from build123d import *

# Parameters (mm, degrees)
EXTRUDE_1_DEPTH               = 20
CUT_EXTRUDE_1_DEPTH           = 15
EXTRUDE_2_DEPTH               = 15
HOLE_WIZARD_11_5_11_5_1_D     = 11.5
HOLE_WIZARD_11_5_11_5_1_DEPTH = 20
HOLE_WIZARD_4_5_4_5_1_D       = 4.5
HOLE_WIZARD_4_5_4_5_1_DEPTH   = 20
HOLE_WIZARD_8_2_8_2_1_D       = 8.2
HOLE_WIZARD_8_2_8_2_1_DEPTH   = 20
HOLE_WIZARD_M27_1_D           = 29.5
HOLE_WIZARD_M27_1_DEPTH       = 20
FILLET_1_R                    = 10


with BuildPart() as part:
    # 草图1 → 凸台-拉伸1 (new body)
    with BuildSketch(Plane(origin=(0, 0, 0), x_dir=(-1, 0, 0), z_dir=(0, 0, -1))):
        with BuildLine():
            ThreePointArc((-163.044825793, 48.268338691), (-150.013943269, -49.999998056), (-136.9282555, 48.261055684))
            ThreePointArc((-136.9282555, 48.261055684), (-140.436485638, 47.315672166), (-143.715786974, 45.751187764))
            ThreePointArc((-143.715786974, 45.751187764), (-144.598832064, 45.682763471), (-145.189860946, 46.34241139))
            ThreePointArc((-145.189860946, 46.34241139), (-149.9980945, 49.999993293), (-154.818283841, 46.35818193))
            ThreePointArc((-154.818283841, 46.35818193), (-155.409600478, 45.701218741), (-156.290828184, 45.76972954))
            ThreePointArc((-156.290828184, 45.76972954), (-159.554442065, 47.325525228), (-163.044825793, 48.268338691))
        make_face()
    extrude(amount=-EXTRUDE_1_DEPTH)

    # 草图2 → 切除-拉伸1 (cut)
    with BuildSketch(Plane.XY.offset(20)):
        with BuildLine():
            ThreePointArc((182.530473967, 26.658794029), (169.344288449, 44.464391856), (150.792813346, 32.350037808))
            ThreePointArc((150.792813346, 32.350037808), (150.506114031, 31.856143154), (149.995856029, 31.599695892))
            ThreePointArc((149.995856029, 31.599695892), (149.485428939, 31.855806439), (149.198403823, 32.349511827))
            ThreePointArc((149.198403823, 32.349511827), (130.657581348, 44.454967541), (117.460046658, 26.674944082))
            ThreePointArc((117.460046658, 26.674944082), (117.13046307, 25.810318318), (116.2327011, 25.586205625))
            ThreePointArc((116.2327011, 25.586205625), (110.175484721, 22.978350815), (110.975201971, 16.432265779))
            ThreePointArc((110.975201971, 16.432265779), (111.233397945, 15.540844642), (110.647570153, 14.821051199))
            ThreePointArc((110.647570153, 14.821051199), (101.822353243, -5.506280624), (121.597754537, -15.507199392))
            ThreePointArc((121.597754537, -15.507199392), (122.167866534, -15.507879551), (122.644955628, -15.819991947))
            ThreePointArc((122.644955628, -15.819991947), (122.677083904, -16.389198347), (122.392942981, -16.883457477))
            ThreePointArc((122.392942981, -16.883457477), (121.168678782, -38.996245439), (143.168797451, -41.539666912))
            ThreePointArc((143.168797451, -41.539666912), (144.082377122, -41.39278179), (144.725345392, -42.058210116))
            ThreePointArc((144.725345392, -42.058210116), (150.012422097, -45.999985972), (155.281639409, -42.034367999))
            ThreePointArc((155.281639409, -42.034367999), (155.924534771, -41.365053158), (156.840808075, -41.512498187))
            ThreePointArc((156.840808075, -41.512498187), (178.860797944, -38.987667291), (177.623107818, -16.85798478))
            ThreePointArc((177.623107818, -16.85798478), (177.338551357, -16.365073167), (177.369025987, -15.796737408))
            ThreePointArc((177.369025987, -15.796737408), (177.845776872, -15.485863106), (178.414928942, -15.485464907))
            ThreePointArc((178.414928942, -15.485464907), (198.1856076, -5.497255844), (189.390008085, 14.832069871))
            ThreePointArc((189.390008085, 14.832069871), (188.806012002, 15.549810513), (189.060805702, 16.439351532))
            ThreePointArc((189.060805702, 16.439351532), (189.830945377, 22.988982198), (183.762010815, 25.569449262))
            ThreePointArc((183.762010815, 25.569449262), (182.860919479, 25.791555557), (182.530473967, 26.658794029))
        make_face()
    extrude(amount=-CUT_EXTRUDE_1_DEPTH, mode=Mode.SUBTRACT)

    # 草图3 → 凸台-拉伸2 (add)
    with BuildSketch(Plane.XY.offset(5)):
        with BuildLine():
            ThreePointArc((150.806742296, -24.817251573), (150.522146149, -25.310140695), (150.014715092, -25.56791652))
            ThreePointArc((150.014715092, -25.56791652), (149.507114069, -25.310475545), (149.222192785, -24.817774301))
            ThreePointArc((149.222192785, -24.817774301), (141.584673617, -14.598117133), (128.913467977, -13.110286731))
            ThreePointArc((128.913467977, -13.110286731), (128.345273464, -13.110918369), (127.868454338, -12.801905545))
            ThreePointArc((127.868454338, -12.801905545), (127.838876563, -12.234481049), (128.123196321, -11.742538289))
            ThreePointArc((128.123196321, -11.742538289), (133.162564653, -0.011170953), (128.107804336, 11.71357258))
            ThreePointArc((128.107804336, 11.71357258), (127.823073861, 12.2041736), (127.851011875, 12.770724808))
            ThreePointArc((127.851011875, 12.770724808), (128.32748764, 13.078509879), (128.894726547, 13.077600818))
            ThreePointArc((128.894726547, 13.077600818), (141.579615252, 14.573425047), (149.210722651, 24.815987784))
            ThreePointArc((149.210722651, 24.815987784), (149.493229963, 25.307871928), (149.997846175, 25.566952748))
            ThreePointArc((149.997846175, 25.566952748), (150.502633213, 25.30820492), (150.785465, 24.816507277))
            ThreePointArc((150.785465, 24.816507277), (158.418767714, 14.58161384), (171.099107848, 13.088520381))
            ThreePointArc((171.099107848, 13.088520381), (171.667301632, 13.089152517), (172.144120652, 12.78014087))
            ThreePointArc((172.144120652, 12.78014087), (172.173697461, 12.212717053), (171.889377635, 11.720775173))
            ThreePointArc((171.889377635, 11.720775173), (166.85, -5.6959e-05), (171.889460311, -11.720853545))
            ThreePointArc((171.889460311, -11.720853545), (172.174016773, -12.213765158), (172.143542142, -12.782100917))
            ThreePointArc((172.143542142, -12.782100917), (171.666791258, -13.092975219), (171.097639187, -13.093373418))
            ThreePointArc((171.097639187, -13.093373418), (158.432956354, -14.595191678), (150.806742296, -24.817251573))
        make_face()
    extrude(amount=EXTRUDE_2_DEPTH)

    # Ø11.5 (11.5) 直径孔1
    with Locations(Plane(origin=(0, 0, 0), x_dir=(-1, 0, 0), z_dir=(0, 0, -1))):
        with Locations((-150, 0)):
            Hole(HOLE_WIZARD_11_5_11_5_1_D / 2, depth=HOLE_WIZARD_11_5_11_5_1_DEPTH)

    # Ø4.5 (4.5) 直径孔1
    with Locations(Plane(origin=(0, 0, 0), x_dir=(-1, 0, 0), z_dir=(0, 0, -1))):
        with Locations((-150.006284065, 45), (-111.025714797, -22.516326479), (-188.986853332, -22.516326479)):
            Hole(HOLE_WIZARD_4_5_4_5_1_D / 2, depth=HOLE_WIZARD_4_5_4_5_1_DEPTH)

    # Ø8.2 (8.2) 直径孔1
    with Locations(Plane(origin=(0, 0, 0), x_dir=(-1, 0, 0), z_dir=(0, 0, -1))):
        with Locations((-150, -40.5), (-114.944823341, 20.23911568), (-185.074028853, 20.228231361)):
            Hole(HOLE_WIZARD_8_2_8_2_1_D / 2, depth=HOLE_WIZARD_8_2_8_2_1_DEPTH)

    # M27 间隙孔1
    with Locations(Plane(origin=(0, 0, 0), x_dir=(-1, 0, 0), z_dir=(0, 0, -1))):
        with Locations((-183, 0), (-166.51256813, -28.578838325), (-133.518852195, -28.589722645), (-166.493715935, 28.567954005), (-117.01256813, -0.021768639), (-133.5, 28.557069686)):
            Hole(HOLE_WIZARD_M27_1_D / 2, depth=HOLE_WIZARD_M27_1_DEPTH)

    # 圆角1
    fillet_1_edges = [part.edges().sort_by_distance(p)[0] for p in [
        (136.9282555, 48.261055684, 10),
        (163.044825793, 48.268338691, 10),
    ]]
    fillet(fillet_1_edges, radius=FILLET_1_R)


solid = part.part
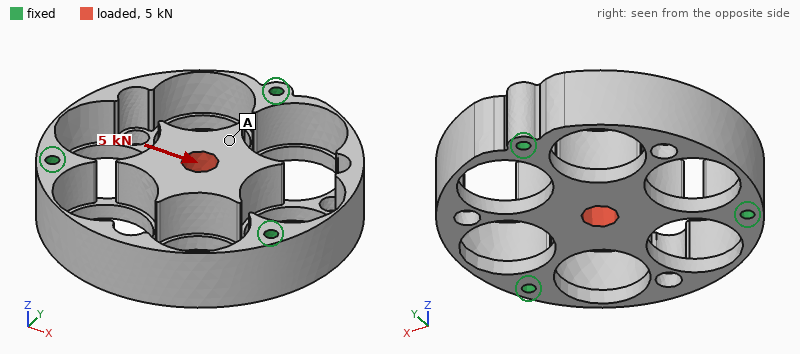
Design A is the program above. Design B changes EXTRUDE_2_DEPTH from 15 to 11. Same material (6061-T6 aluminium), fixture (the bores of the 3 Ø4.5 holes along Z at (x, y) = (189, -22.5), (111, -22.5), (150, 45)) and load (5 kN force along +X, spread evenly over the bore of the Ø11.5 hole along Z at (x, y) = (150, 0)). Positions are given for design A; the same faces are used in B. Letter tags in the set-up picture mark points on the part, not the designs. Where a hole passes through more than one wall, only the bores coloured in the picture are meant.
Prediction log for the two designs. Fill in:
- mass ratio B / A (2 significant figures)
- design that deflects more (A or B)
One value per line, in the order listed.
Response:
0.92
A
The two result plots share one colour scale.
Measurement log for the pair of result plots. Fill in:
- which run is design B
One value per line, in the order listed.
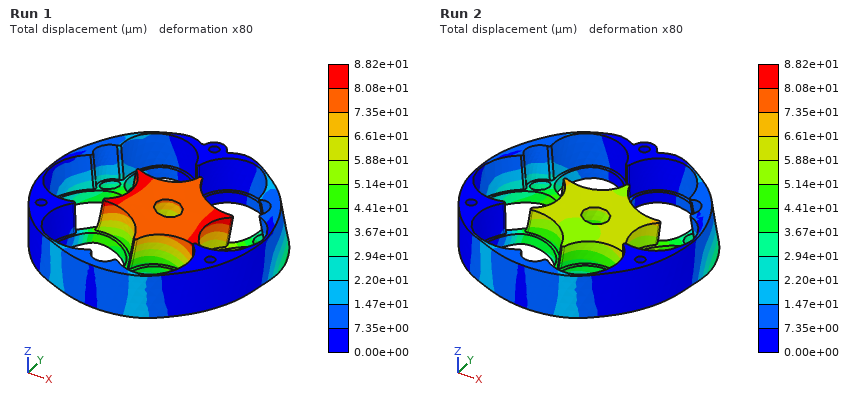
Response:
Run 2
